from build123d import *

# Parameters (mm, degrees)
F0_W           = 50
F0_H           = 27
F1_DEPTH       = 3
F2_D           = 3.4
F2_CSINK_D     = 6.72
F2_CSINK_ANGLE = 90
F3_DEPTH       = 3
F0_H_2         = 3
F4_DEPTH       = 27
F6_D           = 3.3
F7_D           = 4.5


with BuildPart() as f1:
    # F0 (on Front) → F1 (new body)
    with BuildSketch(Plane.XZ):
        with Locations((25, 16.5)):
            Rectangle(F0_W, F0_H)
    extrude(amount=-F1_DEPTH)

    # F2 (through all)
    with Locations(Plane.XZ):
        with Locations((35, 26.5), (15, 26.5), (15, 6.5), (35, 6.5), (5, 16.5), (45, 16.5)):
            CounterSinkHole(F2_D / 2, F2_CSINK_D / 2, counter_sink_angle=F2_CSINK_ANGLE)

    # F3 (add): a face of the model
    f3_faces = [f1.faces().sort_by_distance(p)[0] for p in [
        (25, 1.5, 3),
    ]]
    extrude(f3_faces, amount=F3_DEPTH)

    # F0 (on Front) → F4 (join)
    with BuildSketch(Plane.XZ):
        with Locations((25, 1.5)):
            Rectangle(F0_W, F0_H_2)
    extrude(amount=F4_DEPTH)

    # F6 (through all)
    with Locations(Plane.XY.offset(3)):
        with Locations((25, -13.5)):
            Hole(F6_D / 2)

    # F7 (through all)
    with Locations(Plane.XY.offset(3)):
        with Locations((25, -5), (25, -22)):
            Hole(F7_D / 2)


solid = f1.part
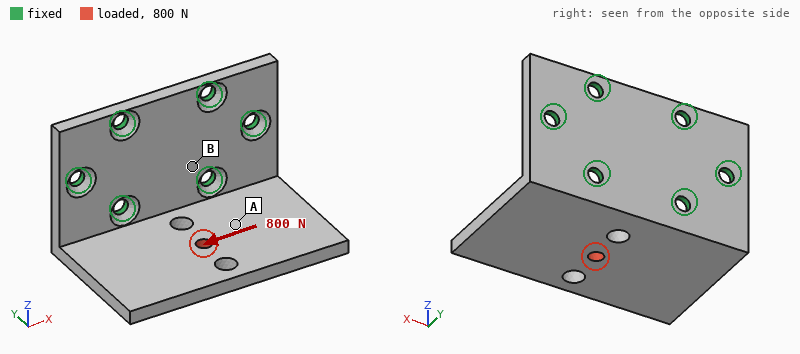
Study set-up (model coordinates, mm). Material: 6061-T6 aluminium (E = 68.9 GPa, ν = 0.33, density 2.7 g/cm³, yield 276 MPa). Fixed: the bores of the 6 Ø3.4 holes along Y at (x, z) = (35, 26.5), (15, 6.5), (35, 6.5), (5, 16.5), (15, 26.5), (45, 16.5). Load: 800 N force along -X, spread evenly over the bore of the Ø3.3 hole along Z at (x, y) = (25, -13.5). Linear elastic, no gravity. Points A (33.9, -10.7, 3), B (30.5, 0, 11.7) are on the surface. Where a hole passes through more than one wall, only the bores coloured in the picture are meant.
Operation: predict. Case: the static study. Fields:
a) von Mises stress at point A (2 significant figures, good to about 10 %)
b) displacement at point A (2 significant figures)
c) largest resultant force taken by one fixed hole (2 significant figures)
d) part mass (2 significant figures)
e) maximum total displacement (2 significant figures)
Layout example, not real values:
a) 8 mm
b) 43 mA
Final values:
a) 21 MPa
b) 27 µm
c) 630 N
d) 22 g
e) 69 µm
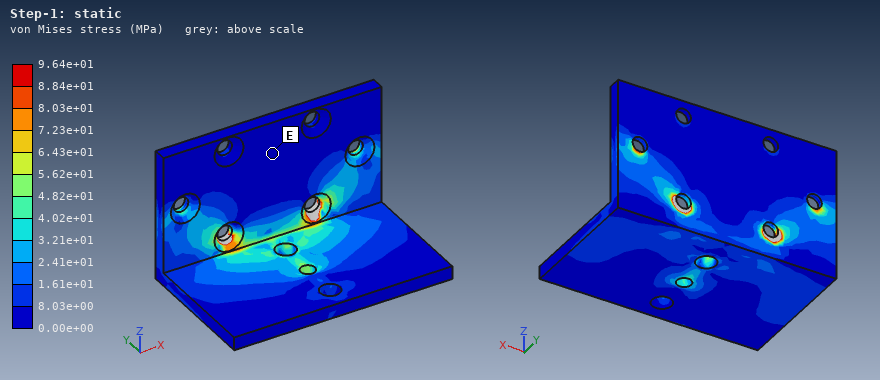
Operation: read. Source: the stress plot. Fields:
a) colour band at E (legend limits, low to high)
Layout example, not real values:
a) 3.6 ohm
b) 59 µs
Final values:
a) 0.00e+00 to 8.03e+00 MPa
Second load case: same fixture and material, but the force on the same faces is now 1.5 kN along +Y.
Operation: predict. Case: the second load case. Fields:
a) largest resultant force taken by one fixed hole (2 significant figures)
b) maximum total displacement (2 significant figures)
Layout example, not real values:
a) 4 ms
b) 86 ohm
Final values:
a) 920 N
b) 0.15 mm
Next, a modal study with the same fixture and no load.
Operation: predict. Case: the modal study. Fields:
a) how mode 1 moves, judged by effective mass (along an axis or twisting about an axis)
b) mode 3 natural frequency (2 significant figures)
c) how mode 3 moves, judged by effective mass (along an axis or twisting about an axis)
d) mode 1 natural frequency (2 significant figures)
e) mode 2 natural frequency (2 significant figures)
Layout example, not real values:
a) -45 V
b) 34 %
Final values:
a) along Z
b) 7100 Hz
c) along X
d) 2200 Hz
e) 3900 Hz
